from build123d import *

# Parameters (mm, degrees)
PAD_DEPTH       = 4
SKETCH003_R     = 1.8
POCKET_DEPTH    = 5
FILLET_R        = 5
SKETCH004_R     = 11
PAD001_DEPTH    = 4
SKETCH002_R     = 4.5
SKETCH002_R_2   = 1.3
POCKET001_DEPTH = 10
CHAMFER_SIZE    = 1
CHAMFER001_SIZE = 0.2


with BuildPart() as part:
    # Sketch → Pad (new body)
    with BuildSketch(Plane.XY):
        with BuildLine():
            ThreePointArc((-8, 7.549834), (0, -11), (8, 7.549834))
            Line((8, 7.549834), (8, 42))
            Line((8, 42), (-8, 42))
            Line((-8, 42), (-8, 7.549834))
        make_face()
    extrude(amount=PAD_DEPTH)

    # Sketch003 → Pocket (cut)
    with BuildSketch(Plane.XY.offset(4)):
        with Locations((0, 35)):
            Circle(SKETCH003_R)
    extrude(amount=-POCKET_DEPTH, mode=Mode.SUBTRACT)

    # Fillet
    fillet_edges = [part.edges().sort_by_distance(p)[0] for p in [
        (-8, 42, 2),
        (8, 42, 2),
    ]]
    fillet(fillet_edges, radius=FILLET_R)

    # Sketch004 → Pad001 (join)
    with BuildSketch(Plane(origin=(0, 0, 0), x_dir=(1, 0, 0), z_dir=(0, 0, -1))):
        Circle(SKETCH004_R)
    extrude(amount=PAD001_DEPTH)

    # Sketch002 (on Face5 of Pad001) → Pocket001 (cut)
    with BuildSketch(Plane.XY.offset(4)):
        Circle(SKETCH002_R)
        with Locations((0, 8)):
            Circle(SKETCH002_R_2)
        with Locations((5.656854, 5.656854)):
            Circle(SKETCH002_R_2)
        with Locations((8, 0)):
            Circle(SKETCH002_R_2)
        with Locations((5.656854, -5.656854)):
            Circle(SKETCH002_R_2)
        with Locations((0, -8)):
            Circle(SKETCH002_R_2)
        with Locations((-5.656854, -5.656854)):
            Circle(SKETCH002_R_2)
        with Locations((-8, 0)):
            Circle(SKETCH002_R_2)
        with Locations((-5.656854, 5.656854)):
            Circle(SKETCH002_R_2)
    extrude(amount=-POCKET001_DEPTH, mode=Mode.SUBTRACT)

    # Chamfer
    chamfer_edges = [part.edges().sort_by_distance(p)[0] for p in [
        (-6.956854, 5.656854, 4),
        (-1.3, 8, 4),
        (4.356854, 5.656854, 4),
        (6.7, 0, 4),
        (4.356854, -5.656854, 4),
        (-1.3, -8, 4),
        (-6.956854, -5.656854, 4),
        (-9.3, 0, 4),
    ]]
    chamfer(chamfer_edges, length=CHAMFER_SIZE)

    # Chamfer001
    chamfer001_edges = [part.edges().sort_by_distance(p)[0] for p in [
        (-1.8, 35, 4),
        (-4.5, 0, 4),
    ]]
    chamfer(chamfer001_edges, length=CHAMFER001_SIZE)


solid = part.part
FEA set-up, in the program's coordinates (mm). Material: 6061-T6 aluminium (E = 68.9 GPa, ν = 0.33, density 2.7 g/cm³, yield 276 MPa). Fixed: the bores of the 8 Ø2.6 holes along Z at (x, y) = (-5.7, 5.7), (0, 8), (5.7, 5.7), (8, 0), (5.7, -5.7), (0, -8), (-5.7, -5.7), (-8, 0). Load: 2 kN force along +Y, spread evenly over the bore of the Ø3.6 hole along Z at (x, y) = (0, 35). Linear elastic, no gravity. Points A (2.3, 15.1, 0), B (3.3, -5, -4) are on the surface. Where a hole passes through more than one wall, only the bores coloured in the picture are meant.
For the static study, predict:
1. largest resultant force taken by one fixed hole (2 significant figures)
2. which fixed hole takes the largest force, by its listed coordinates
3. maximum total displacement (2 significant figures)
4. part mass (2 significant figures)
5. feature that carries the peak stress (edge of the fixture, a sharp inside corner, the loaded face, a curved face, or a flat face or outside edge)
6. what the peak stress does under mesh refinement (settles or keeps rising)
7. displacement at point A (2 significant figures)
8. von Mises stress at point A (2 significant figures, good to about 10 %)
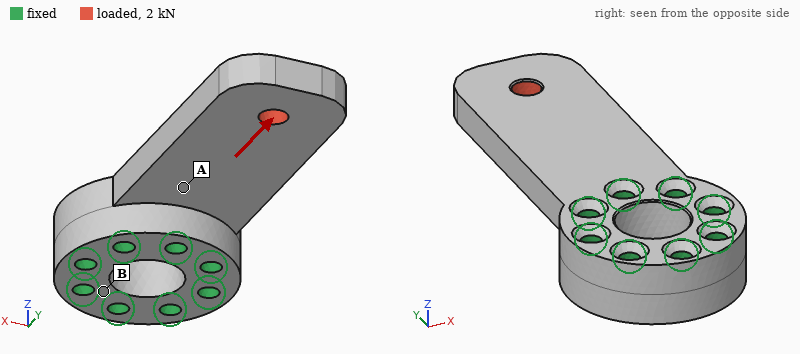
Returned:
820 N
(0, 8)
18 µm
11 g
edge of the fixture
keeps rising
3.6 µm
38 MPa
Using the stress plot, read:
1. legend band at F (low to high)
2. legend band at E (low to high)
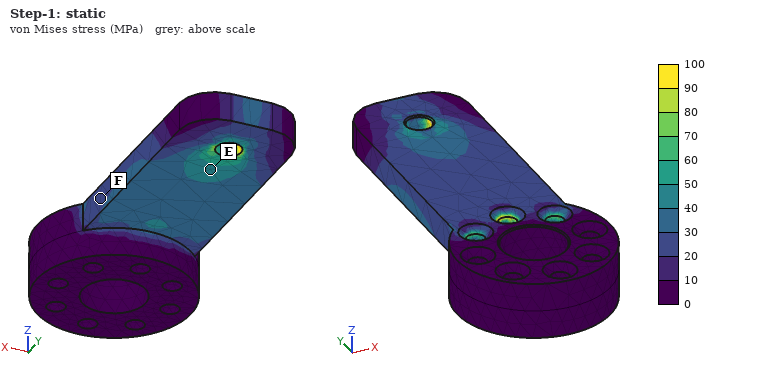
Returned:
20 to 30 MPa
40 to 50 MPa
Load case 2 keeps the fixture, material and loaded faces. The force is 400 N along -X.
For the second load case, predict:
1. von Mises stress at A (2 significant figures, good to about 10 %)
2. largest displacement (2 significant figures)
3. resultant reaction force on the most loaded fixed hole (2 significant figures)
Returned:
23 MPa
54 µm
770 N
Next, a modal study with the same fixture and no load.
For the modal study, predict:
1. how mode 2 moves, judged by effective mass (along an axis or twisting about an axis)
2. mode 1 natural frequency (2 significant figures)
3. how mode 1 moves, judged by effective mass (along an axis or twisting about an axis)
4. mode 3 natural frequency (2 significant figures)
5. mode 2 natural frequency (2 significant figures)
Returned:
along X
3100 Hz
along Z
12 kHz
9600 Hz
